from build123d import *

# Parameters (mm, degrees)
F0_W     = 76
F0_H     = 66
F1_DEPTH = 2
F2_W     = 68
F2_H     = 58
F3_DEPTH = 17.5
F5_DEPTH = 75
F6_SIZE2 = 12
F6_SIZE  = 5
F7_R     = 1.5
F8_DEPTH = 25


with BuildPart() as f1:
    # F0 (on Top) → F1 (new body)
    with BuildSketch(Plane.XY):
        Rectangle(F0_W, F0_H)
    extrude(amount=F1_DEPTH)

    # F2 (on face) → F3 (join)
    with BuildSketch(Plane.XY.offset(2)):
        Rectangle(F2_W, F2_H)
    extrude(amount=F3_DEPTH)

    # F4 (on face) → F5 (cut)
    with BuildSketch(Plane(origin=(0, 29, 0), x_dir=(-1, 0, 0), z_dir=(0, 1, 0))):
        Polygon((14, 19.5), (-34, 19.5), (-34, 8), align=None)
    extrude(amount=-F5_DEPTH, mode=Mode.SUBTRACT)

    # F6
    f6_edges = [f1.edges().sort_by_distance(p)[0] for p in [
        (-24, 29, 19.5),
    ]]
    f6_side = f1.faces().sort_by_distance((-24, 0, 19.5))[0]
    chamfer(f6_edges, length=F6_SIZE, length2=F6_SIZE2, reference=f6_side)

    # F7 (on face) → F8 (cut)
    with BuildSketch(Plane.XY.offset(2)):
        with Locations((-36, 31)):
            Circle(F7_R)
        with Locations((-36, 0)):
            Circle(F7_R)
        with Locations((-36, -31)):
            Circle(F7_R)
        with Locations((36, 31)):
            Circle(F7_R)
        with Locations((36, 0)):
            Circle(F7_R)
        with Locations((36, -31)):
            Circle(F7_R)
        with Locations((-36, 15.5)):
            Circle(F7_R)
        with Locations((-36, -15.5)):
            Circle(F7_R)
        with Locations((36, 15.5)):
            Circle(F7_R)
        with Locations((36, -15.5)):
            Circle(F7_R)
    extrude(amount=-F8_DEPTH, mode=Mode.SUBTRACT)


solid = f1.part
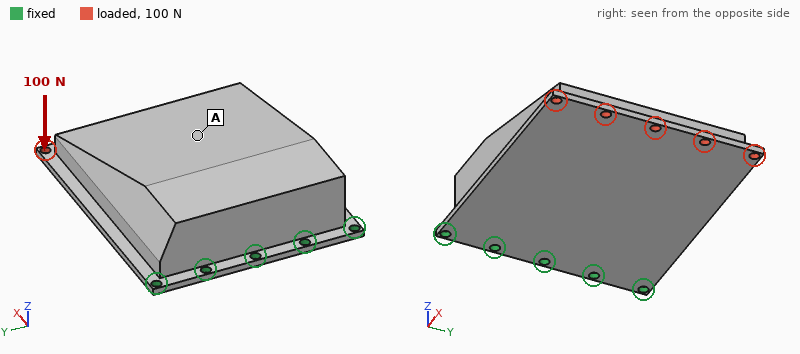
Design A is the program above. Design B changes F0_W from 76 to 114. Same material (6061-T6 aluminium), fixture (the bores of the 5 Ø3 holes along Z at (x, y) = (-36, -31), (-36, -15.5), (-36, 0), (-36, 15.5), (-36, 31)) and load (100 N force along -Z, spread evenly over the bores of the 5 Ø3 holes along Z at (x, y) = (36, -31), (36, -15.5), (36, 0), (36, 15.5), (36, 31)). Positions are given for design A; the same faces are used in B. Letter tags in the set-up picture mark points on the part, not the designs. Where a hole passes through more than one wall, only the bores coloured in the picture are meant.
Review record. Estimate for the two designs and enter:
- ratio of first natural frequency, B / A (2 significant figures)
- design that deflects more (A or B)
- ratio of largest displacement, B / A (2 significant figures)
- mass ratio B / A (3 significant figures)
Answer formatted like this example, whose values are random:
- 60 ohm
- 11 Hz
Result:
- 0.97
- B
- 1.1
- 1.08
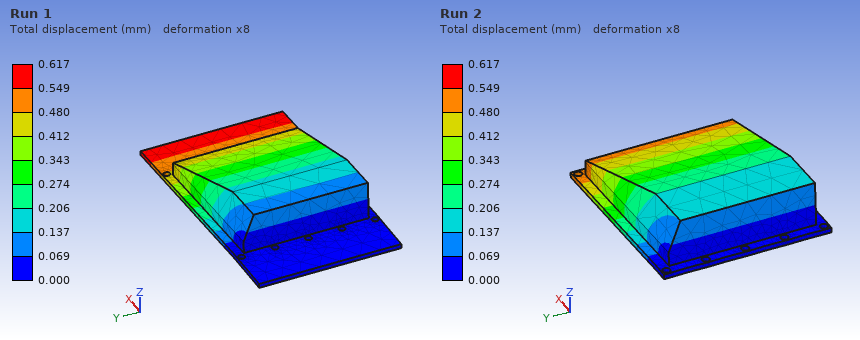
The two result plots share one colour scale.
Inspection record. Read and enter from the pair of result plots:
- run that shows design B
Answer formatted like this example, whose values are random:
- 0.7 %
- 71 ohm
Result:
- Run 1
